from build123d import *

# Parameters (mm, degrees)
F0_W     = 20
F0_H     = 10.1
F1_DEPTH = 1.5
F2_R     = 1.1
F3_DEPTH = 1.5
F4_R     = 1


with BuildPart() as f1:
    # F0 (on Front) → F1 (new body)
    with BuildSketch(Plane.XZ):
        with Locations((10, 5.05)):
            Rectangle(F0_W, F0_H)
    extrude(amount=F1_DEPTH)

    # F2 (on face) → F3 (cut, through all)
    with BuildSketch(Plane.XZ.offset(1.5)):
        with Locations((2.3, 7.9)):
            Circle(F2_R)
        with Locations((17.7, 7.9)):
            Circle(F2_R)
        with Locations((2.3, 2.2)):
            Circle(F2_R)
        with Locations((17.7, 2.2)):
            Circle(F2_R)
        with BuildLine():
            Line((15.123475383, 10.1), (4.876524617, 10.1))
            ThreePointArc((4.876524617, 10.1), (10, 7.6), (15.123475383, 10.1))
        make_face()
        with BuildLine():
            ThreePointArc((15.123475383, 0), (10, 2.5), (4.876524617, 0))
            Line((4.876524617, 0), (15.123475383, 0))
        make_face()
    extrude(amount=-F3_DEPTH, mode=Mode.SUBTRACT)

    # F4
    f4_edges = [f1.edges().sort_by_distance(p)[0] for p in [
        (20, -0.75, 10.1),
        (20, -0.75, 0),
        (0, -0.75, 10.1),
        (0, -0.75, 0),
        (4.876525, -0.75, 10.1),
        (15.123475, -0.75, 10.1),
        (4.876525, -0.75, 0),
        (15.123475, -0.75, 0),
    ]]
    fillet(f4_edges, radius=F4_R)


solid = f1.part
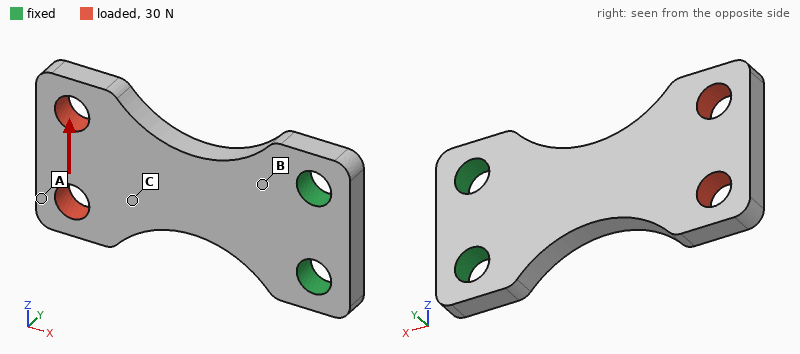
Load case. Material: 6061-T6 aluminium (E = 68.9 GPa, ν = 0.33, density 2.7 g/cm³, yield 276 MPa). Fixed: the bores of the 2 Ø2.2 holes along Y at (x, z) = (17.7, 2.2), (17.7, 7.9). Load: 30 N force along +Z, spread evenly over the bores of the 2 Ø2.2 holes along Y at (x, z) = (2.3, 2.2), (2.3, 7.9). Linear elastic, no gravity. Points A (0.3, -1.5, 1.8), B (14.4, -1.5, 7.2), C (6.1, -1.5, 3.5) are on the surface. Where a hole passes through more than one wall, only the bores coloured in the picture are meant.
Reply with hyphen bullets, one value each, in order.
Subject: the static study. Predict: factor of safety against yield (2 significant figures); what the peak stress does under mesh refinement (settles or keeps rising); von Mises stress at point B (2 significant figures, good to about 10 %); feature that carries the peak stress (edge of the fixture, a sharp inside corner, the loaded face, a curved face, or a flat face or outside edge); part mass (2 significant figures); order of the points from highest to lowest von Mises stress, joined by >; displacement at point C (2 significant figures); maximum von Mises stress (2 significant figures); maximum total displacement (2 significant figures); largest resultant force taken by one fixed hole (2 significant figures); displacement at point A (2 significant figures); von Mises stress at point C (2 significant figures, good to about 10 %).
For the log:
- 6.2
- settles
- 16 MPa
- a curved face
- 0.61 g
- B > C > A
- 8.6 µm
- 44 MPa
- 19 µm
- 69 N
- 18 µm
- 9.8 MPa
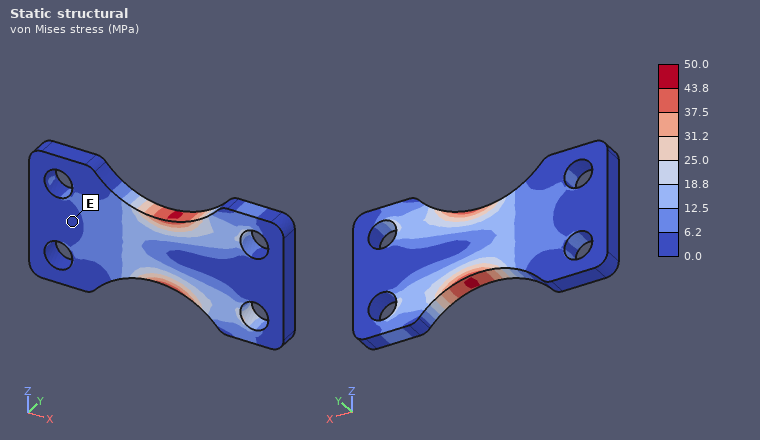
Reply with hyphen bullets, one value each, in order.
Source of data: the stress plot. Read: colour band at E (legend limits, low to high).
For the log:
- 0.0 to 6.2 MPa
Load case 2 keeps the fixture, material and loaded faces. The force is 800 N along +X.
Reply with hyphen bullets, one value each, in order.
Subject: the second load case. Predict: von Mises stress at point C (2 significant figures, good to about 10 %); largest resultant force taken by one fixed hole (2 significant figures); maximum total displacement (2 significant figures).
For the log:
- 70 MPa
- 420 N
- 22 µm
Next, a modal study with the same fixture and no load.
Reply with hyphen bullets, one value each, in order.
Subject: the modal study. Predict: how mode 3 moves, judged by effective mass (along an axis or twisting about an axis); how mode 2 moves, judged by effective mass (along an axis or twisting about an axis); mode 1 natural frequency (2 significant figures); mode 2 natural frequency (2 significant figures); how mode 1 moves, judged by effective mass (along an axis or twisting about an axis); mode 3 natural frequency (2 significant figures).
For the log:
- along Z
- twisting about X
- 4000 Hz
- 14 kHz
- along Y
- 15 kHz
